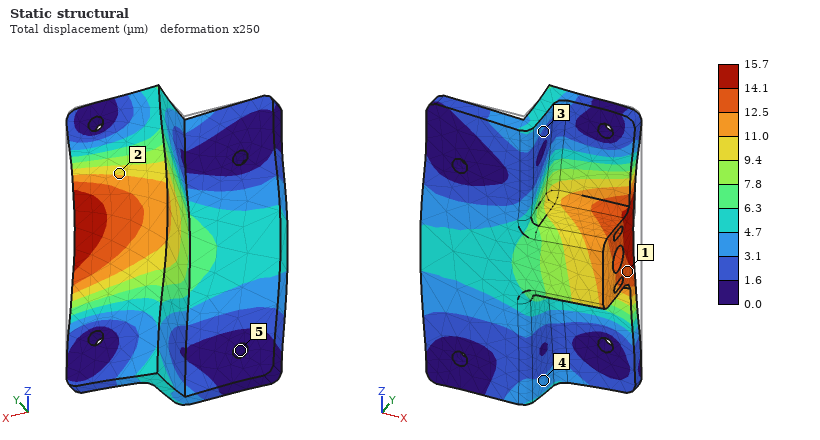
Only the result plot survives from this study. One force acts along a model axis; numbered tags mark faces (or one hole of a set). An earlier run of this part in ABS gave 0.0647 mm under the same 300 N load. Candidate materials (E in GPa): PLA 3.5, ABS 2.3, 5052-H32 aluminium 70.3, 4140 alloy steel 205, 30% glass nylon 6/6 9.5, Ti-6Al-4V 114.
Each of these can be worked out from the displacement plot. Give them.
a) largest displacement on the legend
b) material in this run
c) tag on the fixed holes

15.7 µm
30% glass nylon 6/6
5
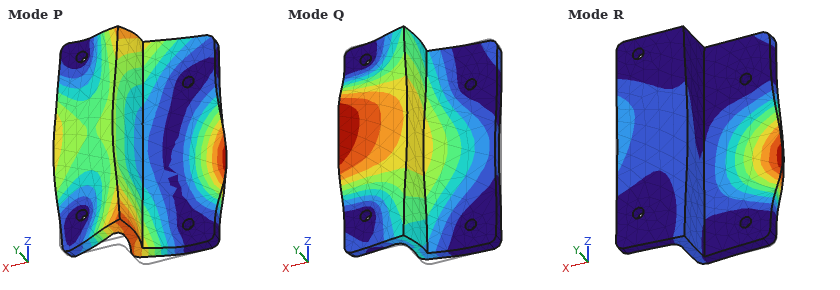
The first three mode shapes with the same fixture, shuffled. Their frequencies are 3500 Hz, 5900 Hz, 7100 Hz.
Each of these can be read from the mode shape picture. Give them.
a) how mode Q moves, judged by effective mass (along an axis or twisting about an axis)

along Y
